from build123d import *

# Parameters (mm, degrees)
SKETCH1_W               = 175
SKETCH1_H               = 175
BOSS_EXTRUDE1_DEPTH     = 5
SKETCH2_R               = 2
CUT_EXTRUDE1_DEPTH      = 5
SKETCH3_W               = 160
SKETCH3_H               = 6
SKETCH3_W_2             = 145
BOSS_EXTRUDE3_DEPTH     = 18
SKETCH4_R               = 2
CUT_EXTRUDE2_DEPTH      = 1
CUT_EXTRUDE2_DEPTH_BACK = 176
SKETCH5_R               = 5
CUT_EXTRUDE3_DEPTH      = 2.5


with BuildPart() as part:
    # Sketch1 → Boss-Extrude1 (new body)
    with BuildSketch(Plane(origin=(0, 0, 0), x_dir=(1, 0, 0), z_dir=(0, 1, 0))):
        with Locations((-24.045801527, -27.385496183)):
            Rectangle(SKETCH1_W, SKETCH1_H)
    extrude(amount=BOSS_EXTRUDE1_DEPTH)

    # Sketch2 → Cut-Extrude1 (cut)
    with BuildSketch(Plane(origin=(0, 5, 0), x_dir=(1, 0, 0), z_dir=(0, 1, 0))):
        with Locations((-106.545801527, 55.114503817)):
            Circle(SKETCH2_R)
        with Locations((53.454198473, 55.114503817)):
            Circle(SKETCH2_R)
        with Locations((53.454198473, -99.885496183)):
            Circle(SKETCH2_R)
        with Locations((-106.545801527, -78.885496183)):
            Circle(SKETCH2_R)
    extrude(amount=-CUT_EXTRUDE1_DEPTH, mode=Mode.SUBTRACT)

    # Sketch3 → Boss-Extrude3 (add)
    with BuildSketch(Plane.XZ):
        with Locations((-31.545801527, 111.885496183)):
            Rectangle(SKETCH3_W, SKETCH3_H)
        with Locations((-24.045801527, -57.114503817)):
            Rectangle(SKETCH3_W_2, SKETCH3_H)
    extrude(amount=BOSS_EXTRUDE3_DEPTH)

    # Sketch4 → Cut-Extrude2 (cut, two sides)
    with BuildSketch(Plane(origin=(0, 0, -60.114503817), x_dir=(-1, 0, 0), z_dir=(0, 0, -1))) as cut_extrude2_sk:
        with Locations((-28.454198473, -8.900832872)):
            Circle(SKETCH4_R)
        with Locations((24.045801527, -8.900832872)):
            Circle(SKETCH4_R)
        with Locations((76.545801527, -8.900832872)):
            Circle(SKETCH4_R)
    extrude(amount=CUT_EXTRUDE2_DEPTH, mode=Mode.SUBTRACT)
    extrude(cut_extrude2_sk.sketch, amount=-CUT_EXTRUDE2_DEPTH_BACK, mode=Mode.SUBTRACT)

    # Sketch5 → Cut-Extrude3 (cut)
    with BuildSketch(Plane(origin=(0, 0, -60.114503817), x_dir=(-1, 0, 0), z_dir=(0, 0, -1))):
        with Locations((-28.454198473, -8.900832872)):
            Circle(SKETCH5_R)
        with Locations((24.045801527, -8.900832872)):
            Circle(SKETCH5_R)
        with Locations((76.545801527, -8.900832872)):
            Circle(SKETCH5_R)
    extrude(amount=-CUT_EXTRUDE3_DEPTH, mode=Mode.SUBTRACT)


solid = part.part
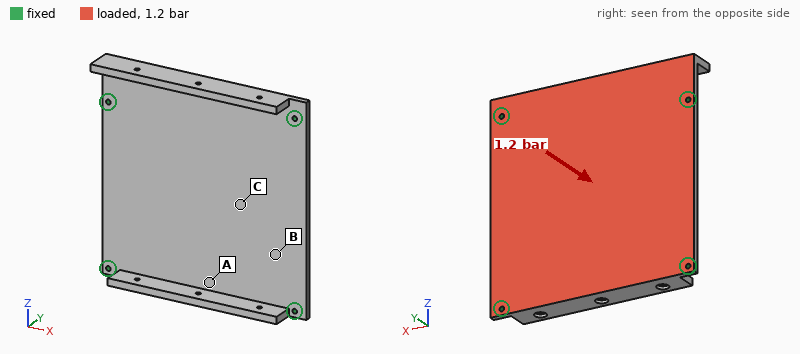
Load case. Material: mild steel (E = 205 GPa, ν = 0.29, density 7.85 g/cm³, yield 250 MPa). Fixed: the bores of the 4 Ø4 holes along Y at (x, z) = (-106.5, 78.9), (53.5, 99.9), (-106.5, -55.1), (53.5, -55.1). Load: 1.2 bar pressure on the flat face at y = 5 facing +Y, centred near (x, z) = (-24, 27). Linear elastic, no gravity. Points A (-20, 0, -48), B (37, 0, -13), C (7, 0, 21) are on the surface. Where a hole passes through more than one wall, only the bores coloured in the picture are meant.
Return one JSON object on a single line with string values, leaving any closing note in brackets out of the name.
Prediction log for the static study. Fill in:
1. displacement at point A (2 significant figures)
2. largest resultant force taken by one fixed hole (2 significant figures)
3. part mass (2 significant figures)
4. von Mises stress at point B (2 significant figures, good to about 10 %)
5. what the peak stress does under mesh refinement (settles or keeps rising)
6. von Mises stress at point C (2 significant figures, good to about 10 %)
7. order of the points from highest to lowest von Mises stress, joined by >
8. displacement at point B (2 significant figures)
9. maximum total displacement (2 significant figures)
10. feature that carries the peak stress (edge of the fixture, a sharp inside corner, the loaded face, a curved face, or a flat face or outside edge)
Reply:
{"displacement at point A": "0.048 mm", "largest resultant force taken by one fixed hole": "1.2 kN", "part mass": "1.5 kg", "von Mises stress at point B": "22 MPa", "what the peak stress does under mesh refinement": "keeps rising", "von Mises stress at point C": "37 MPa", "order of the points from highest to lowest von Mises stress, joined by >": "C > B > A", "displacement at point B": "0.12 mm", "maximum total displacement": "0.19 mm", "feature that carries the peak stress": "edge of the fixture"}
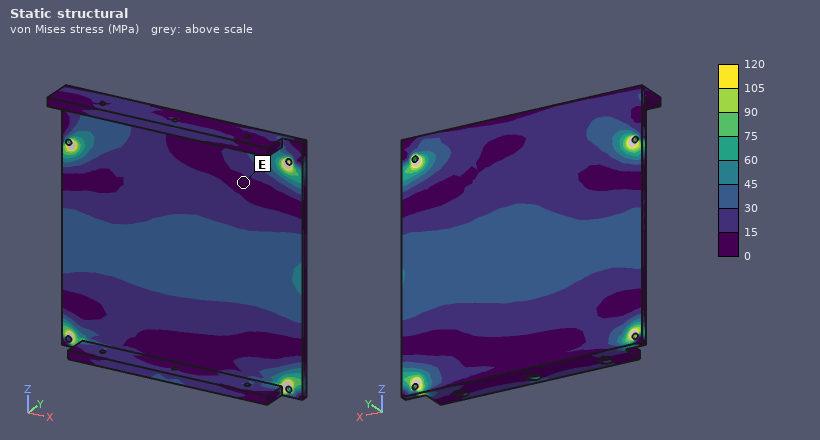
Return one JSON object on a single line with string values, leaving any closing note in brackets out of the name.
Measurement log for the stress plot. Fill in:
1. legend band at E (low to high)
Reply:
{"legend band at E": "0 to 15 MPa"}
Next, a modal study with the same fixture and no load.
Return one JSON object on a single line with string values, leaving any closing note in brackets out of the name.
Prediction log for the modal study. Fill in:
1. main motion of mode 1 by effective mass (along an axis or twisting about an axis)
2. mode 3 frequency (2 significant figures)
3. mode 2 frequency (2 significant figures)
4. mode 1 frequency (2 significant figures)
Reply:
{"main motion of mode 1 by effective mass": "along Y", "mode 3 frequency": "1300 Hz", "mode 2 frequency": "1200 Hz", "mode 1 frequency": "760 Hz"}
